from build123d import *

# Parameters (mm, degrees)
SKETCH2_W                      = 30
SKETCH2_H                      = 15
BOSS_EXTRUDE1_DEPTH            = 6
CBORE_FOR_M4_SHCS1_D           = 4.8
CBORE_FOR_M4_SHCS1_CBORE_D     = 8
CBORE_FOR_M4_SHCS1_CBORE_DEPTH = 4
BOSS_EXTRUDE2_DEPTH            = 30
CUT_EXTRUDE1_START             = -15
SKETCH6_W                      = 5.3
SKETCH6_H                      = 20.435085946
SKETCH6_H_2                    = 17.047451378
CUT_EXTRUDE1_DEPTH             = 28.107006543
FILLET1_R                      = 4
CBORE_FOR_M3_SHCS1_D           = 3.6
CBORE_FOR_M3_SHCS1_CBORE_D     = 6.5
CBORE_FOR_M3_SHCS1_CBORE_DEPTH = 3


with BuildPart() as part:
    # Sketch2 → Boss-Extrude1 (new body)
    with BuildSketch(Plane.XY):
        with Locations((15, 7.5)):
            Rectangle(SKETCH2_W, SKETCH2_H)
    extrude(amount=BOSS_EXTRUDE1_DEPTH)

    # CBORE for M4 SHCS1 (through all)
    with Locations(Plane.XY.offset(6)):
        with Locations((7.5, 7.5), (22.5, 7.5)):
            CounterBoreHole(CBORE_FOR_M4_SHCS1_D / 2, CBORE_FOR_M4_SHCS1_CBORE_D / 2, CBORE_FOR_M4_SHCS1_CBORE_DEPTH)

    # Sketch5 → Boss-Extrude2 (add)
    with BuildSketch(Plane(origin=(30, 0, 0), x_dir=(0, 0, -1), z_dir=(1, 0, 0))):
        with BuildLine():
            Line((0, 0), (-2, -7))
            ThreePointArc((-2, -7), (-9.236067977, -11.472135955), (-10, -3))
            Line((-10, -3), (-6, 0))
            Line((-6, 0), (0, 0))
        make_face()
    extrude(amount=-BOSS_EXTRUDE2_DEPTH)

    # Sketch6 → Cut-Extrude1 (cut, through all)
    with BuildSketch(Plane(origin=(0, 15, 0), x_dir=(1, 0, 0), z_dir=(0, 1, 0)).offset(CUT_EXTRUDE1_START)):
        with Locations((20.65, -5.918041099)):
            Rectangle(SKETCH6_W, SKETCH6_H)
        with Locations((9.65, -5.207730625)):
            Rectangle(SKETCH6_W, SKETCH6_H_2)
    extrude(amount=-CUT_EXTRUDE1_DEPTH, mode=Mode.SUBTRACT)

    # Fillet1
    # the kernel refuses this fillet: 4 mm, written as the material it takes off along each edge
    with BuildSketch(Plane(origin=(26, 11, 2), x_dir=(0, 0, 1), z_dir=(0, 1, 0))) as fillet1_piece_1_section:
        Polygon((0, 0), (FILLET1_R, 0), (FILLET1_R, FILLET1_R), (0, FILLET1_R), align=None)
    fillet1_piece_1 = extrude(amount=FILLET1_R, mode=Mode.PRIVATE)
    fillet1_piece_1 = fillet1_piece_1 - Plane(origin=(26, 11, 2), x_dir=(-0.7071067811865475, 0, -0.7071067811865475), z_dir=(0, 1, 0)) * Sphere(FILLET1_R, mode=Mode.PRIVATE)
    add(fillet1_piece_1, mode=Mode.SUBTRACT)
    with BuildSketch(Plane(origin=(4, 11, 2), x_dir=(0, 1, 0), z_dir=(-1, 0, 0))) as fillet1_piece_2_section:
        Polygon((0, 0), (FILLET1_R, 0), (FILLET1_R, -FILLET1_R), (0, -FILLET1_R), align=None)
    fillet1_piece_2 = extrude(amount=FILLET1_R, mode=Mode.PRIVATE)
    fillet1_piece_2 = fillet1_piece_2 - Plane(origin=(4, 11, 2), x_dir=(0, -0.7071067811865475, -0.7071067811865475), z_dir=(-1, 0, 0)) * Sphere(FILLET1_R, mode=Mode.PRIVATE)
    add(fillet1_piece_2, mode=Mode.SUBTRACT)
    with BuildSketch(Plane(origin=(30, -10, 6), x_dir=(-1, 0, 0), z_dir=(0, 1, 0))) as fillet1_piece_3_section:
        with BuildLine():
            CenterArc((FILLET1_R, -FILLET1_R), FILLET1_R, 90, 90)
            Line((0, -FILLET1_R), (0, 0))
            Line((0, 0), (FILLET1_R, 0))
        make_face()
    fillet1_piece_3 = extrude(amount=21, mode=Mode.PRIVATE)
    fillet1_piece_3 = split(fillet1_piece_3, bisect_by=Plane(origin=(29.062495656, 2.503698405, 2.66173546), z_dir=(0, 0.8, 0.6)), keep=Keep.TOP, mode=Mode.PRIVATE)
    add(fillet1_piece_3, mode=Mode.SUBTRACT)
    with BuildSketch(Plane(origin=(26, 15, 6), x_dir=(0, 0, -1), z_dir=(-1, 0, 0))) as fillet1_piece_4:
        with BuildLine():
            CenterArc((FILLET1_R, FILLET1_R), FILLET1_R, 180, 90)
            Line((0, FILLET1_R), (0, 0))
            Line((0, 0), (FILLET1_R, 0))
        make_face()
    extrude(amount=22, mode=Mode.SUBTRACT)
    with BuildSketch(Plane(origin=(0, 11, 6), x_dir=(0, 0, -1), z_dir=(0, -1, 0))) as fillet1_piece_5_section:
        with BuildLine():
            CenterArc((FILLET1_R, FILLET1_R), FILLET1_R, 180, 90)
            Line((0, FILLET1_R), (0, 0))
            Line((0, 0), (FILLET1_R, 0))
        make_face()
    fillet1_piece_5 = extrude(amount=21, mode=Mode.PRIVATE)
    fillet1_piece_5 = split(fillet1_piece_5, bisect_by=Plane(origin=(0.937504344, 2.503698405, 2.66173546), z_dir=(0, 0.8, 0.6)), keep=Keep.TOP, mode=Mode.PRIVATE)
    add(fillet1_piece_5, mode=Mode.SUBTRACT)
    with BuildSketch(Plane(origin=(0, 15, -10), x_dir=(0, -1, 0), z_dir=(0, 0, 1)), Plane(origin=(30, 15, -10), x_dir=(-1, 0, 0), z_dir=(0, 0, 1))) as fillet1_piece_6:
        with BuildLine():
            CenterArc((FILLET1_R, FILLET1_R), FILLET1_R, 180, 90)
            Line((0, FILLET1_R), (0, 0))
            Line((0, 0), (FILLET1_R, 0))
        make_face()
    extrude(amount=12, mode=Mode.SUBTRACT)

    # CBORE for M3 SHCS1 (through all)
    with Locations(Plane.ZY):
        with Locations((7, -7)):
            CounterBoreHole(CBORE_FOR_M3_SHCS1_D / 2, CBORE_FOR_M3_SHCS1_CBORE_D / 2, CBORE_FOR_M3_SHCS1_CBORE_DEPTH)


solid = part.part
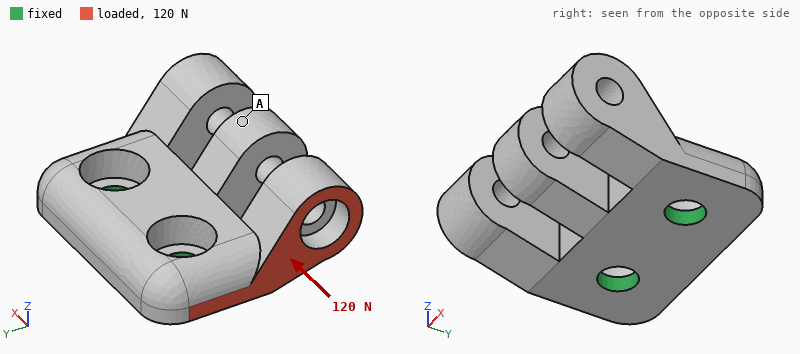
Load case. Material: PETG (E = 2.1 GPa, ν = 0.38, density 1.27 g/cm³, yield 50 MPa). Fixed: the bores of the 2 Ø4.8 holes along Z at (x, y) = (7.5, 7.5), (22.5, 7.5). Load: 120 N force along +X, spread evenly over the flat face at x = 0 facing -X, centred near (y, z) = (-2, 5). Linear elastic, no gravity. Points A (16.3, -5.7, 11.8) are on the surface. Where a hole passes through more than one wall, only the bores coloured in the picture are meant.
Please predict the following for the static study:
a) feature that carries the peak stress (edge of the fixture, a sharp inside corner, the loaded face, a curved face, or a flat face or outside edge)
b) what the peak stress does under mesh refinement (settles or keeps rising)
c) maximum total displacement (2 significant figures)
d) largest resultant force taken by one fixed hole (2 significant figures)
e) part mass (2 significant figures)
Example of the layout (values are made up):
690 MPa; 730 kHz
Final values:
a sharp inside corner; keeps rising; 0.30 mm; 86 N; 4.7 g
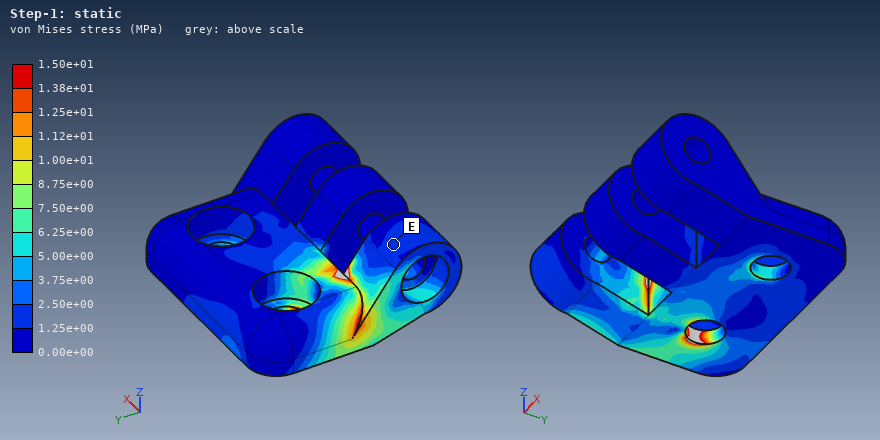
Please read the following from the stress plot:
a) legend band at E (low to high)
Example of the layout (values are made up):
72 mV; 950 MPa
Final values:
1.25e+00 to 2.50e+00 MPa
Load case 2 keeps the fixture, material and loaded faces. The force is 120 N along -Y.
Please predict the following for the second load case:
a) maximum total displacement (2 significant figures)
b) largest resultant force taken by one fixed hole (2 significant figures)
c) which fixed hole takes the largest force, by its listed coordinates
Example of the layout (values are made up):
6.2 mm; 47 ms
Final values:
0.49 mm; 150 N; (7.5, 7.5)
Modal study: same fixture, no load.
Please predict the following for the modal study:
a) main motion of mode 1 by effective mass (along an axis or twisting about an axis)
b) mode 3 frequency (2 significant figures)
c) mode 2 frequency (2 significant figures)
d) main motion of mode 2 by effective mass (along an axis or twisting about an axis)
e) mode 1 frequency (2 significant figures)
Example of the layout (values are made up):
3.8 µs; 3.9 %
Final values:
along Z; 3100 Hz; 2100 Hz; twisting about Y; 1700 Hz
